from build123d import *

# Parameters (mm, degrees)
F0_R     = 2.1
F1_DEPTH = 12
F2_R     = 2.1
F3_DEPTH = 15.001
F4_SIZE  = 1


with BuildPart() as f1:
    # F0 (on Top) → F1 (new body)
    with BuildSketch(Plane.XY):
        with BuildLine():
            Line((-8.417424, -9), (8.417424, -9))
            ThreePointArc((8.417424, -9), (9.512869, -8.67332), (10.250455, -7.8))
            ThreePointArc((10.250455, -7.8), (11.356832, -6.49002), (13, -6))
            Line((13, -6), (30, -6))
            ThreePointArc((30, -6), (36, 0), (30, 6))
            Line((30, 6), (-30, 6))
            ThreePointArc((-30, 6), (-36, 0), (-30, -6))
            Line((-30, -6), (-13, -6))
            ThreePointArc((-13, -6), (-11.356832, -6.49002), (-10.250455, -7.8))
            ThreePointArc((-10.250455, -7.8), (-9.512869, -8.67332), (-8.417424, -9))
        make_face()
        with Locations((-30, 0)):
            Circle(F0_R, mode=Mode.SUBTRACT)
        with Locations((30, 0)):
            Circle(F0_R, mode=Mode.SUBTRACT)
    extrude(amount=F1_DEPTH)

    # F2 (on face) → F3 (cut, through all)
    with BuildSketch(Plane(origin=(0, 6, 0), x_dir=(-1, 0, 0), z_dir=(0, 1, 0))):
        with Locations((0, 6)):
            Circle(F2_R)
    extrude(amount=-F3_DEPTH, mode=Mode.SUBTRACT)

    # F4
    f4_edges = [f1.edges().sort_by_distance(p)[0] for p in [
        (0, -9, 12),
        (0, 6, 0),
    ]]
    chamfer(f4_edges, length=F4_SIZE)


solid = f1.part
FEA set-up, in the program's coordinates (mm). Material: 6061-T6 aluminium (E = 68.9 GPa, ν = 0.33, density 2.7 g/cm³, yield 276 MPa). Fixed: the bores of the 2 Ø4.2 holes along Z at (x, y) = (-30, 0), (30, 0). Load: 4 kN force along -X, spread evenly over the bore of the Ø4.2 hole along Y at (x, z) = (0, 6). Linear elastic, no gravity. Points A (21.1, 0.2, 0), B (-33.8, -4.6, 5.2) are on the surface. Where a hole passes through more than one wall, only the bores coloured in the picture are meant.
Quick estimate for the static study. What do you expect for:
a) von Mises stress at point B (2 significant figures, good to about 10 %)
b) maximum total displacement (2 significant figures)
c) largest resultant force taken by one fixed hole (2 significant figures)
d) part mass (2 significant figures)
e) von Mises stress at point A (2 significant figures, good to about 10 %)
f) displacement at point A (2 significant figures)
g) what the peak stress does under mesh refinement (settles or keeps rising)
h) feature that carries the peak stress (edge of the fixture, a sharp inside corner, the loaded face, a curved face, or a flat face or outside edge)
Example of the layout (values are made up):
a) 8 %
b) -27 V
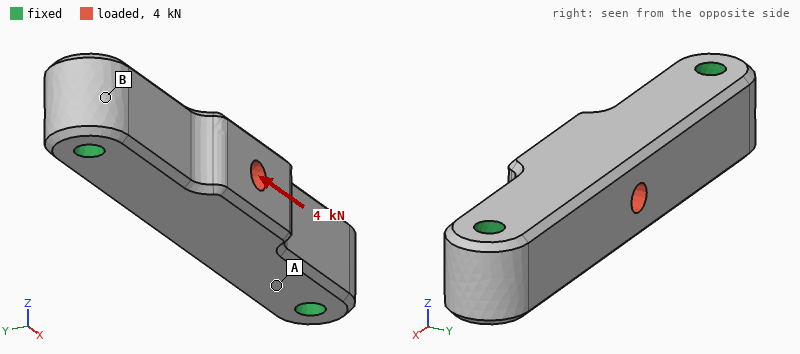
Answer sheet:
a) 3.4 MPa
b) 6.8 µm
c) 2.0 kN
d) 27 g
e) 16 MPa
f) 2.0 µm
g) keeps rising
h) edge of the fixture
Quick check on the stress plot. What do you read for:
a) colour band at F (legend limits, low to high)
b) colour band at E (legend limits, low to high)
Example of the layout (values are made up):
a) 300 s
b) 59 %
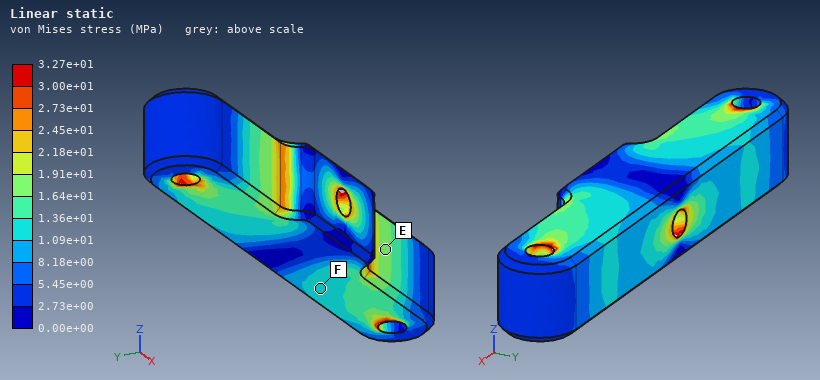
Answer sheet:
a) 1.09e+01 to 1.36e+01 MPa
b) 1.64e+01 to 1.91e+01 MPa
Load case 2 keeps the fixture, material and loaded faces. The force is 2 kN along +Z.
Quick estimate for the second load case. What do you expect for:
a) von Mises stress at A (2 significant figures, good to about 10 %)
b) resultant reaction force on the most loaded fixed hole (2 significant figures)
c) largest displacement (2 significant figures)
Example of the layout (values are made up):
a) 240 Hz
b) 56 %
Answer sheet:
a) 23 MPa
b) 1.0 kN
c) 30 µm
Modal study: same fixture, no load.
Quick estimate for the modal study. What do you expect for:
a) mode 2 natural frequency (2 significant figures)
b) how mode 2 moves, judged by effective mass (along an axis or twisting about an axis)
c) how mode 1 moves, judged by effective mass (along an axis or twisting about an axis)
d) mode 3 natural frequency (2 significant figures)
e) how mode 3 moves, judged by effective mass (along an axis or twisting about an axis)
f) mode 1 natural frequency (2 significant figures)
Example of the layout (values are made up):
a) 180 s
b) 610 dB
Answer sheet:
a) 14 kHz
b) along Z
c) along Y
d) 22 kHz
e) twisting about X
f) 12 kHz
